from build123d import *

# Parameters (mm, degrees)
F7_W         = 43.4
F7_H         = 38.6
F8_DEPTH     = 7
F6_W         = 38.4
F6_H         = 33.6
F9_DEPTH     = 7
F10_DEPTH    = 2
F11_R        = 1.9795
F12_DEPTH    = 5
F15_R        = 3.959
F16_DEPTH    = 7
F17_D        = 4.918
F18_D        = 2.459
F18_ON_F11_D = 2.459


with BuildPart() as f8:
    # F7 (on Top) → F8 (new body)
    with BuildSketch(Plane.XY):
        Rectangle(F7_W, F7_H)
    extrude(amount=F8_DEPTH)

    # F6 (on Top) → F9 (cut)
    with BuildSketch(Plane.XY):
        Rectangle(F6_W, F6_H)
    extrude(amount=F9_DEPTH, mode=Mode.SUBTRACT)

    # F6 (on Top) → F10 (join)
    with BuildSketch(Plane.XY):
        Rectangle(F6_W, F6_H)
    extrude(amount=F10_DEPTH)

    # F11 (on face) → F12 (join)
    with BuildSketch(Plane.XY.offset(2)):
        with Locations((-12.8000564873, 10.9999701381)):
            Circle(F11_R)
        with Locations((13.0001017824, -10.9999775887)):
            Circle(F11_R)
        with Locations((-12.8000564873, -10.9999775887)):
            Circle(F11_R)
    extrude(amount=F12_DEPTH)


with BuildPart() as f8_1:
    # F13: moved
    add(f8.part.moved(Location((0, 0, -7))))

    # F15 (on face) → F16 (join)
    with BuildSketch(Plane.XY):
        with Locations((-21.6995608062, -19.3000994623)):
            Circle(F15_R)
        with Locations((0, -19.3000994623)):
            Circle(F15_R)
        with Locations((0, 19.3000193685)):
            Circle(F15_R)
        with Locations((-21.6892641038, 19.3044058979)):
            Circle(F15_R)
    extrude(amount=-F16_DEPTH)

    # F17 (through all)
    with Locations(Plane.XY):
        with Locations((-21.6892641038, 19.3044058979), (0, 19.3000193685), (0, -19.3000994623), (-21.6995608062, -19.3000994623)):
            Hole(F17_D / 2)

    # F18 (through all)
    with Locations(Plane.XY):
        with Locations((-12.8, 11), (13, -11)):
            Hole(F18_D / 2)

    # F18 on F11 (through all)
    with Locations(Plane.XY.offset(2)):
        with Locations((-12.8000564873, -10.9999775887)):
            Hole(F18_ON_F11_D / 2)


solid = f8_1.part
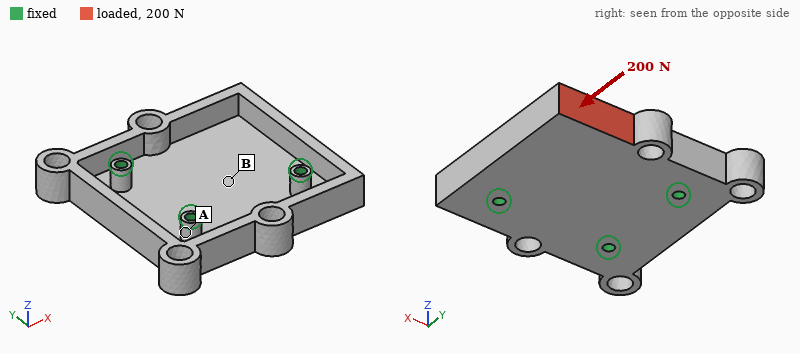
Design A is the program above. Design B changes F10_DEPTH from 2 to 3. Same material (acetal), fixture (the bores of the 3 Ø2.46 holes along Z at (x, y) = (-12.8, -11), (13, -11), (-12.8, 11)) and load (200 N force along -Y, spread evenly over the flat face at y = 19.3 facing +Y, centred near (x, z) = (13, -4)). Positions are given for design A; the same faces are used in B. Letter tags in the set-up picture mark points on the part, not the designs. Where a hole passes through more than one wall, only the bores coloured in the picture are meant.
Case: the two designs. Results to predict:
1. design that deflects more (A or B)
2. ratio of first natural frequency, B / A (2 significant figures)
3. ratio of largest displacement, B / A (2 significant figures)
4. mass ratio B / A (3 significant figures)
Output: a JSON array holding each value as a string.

["A", "1.4", "0.41", "1.22"]
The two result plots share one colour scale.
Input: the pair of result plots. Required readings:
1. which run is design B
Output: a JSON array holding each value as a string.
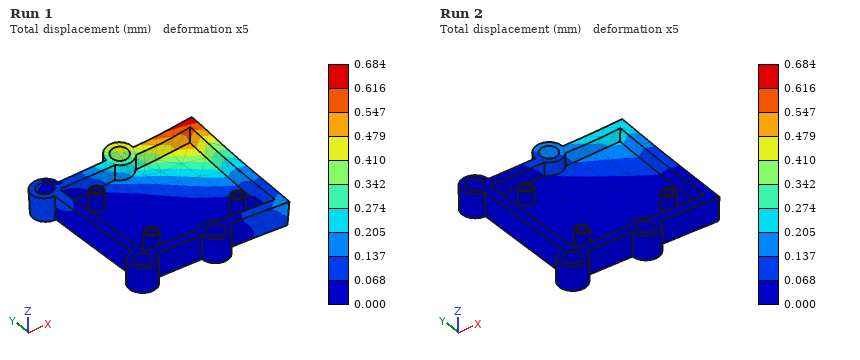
["Run 2"]
